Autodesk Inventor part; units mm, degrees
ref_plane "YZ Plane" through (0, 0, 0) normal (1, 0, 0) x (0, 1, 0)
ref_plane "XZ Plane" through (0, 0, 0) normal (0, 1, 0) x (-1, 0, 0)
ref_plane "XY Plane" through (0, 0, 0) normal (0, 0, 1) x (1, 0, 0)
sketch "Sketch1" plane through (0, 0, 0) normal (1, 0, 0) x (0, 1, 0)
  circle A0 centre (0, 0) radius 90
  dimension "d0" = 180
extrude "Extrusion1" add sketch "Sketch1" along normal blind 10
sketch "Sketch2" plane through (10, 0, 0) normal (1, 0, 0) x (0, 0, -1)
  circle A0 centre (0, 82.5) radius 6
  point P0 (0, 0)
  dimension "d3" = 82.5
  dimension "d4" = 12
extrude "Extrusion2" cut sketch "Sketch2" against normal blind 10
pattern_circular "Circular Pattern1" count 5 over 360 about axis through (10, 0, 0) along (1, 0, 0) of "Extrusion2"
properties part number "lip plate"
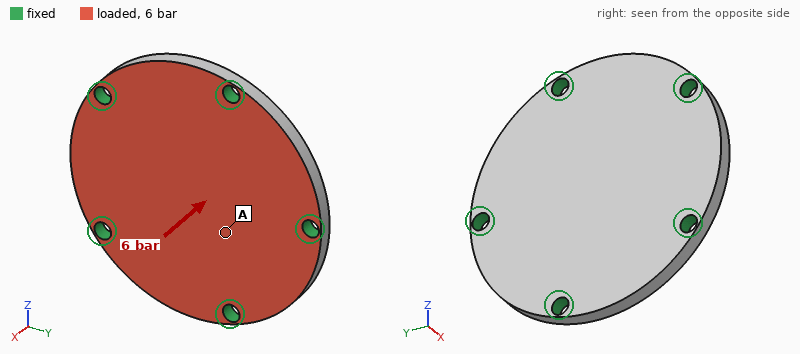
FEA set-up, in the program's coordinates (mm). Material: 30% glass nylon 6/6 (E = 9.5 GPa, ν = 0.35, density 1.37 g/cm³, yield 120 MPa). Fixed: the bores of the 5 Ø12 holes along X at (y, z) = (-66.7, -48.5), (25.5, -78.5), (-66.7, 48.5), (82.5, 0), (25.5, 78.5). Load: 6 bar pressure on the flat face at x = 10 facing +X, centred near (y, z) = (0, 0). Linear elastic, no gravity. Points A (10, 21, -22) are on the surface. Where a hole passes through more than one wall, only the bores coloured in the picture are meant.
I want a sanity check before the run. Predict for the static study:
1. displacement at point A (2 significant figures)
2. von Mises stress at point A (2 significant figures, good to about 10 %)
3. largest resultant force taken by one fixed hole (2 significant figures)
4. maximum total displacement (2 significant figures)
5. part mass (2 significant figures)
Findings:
0.56 mm
18 MPa
3.0 kN
0.69 mm
340 g
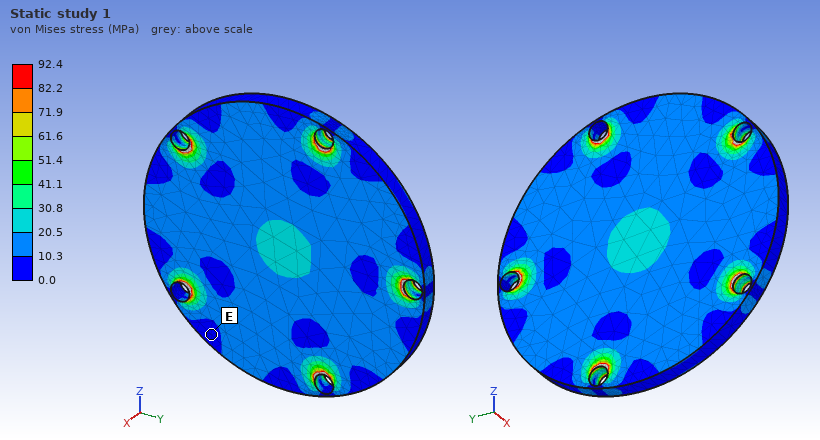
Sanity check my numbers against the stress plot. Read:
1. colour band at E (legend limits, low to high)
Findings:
0.0 to 10.3 MPa
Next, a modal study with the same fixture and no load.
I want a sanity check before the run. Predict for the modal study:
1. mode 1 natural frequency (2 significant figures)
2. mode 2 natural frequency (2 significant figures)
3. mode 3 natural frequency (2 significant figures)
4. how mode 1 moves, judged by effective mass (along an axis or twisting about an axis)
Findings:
1600 Hz
2700 Hz
2700 Hz
along X
